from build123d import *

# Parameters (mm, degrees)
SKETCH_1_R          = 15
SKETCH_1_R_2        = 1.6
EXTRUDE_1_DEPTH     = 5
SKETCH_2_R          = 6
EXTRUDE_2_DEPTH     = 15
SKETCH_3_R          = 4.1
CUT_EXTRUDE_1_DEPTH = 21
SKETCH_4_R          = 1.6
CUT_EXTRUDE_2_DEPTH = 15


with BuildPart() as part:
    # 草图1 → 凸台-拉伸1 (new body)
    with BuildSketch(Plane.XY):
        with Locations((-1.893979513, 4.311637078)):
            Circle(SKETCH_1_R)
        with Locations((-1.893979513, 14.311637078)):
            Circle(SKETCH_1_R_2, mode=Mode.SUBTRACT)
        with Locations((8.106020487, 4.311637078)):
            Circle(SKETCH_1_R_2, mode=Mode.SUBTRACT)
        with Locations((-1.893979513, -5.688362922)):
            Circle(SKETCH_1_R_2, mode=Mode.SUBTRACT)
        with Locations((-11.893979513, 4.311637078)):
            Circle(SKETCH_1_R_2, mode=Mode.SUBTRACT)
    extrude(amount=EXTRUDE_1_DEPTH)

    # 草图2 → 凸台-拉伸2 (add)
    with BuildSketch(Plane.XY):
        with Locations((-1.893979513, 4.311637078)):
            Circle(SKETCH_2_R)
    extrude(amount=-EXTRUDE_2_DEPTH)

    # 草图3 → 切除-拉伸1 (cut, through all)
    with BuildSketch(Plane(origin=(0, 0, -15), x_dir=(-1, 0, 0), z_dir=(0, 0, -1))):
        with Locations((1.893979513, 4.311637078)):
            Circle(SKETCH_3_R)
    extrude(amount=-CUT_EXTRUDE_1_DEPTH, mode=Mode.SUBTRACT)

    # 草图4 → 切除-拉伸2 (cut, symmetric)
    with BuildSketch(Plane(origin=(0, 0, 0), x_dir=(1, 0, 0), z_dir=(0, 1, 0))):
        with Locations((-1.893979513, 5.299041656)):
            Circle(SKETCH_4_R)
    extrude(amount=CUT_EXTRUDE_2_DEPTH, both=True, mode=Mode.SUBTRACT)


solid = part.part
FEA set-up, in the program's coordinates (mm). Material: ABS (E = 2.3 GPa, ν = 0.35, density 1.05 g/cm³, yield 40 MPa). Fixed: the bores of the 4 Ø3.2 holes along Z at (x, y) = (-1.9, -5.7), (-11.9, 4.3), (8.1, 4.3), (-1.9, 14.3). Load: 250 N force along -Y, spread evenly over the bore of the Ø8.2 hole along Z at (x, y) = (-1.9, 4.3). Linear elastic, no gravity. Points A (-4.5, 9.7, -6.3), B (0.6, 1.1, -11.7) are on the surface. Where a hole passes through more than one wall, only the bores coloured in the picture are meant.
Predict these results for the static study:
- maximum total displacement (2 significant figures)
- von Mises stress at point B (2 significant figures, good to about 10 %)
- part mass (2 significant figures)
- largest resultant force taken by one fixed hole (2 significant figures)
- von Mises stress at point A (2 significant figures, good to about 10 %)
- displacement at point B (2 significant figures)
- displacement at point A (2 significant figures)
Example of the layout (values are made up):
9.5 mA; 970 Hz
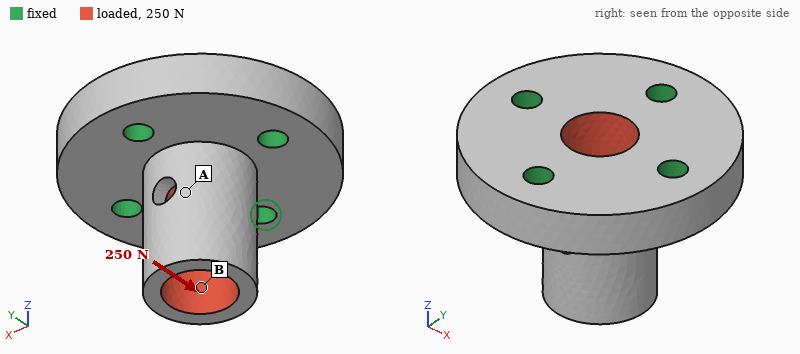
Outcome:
0.17 mm; 2.2 MPa; 4.2 g; 130 N; 6.2 MPa; 0.13 mm; 0.085 mm
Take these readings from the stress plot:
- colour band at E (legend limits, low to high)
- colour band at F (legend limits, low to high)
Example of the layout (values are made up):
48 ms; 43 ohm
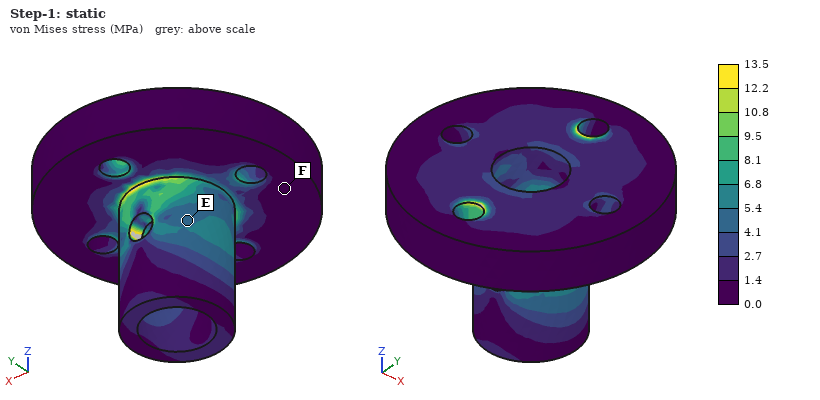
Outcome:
4.1 to 5.4 MPa; 0.0 to 1.4 MPa
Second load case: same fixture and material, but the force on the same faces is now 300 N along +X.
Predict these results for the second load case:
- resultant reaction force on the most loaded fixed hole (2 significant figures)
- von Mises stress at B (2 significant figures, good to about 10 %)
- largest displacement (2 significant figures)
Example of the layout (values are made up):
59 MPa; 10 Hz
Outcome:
160 N; 3.3 MPa; 0.20 mm
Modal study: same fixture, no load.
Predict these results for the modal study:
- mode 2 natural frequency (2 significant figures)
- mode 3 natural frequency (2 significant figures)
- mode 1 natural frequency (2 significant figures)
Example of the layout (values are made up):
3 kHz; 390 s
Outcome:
6500 Hz; 13 kHz; 6400 Hz
